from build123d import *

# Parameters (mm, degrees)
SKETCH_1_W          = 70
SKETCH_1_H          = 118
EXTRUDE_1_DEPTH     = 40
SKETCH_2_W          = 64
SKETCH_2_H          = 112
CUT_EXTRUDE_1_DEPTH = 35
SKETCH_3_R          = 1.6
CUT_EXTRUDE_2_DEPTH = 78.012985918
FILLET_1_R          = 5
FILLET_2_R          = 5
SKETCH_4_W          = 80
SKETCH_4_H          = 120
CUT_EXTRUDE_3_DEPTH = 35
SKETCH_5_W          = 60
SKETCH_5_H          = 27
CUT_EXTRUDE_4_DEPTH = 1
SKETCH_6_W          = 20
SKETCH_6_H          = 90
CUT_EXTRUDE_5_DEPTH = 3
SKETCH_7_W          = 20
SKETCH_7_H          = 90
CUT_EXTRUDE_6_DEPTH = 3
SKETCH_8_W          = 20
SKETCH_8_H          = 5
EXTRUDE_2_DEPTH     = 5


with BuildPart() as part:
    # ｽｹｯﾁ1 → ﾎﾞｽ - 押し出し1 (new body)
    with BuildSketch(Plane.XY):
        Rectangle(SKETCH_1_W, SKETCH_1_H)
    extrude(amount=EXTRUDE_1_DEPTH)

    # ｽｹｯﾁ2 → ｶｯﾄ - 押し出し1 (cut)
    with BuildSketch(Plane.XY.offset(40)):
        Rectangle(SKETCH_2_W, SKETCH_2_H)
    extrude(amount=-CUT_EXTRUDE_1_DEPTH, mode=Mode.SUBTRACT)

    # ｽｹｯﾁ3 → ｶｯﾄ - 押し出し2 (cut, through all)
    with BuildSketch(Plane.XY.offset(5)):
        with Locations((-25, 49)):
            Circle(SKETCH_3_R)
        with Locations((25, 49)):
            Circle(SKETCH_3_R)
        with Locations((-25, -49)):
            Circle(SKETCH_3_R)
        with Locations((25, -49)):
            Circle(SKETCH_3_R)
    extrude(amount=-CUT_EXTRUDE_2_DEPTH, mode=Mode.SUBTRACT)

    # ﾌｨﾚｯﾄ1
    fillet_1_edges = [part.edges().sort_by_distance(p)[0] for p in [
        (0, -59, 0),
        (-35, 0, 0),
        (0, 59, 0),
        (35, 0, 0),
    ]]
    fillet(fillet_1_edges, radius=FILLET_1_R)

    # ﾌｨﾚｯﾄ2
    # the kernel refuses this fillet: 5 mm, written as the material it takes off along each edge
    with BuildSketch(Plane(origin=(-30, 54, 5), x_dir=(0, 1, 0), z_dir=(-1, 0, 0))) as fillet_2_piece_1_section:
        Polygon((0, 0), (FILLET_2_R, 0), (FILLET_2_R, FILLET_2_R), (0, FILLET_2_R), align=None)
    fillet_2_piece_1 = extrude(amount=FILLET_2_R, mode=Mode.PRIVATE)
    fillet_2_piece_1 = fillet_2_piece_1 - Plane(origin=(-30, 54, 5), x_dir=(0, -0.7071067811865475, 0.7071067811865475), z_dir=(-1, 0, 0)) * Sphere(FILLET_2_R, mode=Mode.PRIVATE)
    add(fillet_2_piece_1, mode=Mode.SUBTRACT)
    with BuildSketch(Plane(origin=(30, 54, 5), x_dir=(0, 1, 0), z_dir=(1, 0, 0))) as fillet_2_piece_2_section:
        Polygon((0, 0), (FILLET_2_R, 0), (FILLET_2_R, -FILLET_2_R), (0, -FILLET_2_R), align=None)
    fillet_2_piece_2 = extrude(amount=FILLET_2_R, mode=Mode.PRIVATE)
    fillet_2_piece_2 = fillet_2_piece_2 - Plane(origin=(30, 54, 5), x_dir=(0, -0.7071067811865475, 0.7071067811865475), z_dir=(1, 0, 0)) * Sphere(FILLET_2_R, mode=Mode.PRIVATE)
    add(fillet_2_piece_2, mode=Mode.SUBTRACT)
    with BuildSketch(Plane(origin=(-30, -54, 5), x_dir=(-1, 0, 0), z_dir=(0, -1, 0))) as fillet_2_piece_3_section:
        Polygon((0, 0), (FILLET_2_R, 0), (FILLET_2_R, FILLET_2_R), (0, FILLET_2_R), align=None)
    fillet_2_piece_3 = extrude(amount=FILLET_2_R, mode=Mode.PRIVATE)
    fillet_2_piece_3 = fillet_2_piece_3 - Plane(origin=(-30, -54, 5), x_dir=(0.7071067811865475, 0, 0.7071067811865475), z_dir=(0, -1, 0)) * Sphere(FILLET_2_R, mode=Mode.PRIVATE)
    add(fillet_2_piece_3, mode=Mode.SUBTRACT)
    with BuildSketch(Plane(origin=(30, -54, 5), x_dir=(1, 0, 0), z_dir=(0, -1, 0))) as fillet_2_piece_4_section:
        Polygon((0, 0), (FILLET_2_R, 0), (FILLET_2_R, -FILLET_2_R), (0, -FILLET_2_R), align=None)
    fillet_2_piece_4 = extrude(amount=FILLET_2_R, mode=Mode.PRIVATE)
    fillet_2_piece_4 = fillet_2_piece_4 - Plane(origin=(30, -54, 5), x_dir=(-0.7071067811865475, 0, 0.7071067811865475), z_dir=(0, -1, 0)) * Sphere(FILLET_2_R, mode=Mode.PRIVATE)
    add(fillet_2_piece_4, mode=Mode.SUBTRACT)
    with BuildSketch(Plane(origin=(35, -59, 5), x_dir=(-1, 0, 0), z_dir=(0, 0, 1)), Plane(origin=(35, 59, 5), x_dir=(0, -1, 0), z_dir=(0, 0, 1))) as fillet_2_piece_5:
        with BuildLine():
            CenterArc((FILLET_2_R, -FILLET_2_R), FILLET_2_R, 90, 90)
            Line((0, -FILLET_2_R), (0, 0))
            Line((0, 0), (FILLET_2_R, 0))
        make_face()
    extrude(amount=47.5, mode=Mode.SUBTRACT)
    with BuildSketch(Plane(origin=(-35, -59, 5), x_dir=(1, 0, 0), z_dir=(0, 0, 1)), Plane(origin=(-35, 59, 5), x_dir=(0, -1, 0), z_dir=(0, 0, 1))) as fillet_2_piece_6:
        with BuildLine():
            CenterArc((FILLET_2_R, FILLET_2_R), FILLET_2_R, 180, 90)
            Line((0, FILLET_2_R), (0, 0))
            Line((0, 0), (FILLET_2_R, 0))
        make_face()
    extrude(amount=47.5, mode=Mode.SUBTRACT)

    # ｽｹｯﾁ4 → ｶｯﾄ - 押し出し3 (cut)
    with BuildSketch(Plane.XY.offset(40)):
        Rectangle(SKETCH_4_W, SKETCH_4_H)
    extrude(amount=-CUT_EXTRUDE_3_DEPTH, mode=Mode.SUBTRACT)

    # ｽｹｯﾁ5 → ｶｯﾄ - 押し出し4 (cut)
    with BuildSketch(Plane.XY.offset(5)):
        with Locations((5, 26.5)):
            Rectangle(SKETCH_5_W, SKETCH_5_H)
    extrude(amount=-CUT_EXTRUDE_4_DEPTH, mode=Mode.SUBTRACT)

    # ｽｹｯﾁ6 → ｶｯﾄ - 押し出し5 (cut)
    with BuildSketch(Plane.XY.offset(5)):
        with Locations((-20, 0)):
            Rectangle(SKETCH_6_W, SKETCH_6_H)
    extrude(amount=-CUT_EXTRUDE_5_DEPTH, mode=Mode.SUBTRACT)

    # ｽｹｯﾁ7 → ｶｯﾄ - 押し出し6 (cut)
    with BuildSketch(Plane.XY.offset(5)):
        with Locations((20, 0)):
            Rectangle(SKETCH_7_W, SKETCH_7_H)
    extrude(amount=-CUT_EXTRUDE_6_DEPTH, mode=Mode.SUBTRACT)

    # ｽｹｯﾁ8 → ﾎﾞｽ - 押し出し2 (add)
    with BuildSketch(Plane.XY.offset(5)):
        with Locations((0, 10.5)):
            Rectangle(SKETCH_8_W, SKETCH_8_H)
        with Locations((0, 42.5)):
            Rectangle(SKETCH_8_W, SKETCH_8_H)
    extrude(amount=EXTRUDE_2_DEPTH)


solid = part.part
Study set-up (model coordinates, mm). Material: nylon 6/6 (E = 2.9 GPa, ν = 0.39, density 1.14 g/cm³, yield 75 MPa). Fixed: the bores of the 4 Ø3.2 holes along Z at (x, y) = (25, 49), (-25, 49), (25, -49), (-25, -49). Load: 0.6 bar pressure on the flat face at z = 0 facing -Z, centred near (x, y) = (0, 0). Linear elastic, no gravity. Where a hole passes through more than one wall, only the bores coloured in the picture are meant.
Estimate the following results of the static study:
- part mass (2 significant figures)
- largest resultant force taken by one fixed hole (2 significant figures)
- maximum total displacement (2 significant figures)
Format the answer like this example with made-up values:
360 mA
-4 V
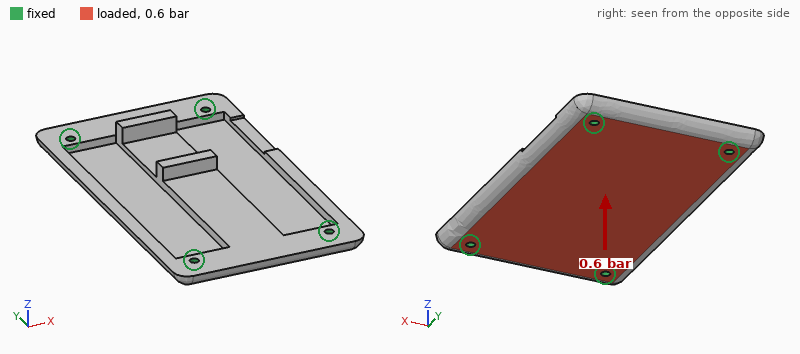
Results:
33 g
98 N
1.3 mm
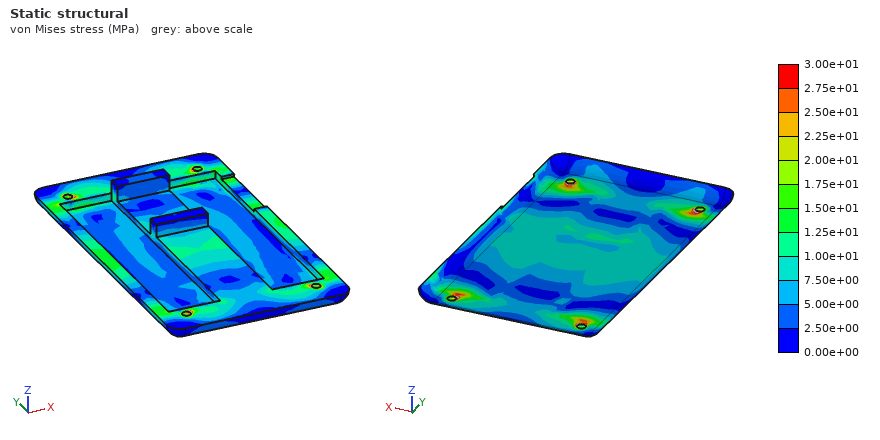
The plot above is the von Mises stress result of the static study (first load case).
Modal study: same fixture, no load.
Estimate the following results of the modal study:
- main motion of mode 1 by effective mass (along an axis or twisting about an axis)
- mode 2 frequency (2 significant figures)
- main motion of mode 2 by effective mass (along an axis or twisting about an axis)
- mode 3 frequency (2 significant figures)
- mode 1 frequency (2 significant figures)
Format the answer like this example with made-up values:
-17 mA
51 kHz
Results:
along Z
900 Hz
twisting about Y
1300 Hz
620 Hz
